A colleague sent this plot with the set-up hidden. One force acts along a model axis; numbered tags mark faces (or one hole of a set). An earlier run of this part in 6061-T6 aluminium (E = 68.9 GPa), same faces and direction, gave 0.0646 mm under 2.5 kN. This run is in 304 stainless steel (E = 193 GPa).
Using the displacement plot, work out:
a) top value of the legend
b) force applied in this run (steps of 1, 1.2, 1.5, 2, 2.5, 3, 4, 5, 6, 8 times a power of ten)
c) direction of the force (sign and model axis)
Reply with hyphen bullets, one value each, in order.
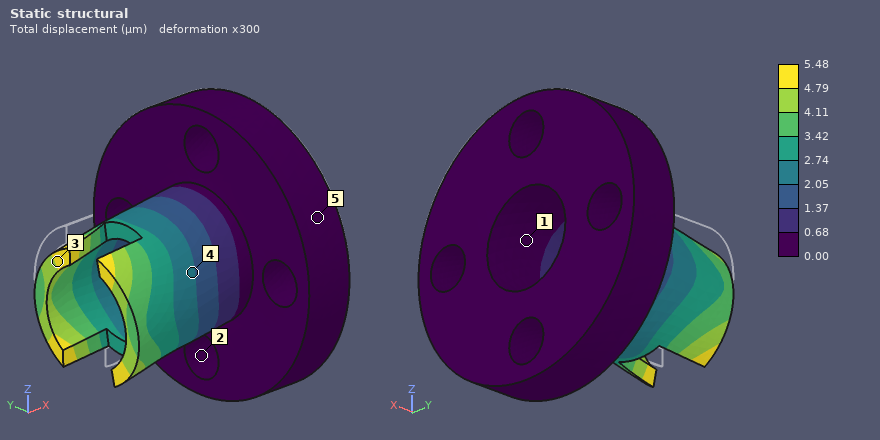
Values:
- 5.48 µm
- 600 N
- -Z
